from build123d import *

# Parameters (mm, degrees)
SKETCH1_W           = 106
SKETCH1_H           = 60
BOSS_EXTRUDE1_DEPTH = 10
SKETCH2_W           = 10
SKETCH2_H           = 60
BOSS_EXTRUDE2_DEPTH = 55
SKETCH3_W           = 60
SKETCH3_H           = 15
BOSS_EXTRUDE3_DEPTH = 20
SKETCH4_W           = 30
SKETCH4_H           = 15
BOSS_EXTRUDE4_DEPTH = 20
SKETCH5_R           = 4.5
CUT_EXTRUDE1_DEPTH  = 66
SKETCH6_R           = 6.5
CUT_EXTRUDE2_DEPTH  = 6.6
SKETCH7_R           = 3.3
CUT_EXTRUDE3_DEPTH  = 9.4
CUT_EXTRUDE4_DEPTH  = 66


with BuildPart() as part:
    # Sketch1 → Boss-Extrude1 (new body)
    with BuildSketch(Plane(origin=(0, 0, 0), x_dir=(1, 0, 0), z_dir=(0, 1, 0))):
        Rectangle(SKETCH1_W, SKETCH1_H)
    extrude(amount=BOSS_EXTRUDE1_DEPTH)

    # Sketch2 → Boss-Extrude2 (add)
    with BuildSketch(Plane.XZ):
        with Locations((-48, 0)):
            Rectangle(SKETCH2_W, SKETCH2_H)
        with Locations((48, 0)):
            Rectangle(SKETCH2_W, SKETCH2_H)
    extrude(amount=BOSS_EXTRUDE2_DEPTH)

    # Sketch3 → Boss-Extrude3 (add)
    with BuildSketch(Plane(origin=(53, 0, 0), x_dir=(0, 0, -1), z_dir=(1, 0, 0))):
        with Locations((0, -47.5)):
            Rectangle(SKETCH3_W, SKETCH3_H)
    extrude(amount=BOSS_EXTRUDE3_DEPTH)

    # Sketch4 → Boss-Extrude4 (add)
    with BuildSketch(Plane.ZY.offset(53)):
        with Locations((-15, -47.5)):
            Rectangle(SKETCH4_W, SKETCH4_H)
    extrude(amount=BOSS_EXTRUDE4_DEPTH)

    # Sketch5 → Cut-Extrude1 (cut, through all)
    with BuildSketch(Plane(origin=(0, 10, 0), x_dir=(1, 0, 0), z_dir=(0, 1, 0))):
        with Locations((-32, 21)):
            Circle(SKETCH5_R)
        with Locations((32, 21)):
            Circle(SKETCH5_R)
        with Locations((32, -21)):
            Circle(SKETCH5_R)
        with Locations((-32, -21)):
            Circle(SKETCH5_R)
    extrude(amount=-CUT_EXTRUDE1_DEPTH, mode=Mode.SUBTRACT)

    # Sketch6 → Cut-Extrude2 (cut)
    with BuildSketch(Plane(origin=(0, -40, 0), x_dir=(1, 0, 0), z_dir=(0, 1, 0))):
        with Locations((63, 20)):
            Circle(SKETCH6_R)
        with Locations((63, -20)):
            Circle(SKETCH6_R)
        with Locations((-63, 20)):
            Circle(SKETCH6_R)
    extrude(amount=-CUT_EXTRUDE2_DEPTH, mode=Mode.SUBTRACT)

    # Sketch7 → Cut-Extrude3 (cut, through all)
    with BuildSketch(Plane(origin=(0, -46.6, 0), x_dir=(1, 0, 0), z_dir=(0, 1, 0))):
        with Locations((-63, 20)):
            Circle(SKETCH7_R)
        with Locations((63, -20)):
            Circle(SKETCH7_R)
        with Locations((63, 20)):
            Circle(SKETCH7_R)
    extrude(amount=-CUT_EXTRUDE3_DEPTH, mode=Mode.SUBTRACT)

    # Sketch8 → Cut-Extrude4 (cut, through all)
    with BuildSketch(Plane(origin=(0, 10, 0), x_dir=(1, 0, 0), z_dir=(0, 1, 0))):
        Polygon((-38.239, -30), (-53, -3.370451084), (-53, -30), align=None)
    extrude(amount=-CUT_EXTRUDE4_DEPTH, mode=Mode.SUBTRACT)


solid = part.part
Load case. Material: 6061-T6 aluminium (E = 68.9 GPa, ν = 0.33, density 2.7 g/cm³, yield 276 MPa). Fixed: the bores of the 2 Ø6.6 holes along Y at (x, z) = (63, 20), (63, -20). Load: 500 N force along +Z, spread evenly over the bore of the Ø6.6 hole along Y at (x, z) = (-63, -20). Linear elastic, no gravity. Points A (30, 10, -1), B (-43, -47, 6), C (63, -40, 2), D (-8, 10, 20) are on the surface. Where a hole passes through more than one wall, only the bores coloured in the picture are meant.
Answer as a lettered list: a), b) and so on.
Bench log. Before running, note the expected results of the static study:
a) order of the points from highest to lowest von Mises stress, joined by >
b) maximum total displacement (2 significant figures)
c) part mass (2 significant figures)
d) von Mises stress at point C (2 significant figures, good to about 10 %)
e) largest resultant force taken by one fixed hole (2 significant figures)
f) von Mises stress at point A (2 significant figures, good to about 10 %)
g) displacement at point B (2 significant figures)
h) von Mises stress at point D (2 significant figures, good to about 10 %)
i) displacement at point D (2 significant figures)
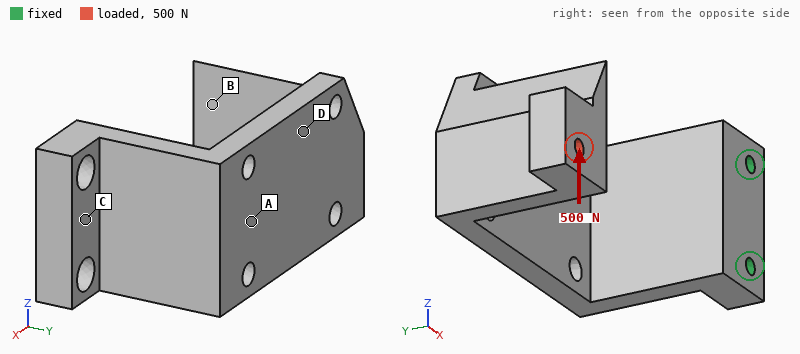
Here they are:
a) A > D > C > B
b) 1.00 mm
c) 380 g
d) 11 MPa
e) 1.4 kN
f) 30 MPa
g) 0.76 mm
h) 23 MPa
i) 0.26 mm
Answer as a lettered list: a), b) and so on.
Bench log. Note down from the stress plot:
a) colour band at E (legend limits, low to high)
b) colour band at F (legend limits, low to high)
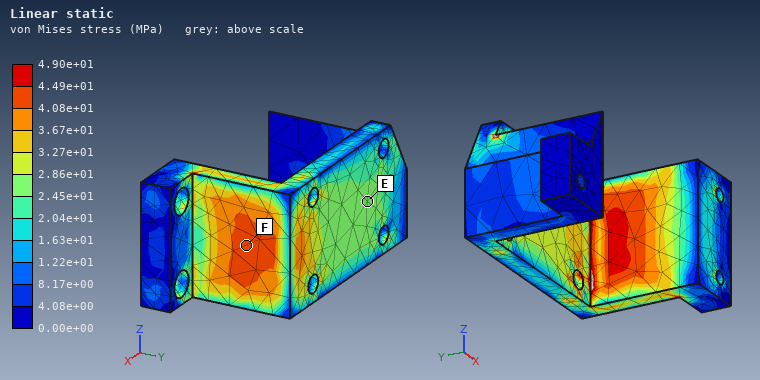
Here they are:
a) 2.45e+01 to 2.86e+01 MPa
b) 4.08e+01 to 4.49e+01 MPa
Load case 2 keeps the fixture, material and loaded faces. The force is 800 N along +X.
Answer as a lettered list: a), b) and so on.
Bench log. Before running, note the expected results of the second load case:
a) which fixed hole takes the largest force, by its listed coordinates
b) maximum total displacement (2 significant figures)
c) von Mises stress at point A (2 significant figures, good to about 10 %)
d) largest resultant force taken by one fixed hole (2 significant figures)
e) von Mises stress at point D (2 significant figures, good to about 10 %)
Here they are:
a) (63, -20)
b) 1.9 mm
c) 48 MPa
d) 760 N
e) 42 MPa
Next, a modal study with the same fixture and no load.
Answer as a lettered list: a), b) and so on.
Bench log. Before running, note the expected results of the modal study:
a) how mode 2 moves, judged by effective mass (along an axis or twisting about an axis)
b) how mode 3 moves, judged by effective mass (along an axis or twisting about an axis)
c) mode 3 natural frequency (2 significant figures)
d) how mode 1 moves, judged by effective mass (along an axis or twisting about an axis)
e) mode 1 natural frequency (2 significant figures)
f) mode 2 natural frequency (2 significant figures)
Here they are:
a) along Z
b) along X
c) 700 Hz
d) along Y
e) 260 Hz
f) 440 Hz
